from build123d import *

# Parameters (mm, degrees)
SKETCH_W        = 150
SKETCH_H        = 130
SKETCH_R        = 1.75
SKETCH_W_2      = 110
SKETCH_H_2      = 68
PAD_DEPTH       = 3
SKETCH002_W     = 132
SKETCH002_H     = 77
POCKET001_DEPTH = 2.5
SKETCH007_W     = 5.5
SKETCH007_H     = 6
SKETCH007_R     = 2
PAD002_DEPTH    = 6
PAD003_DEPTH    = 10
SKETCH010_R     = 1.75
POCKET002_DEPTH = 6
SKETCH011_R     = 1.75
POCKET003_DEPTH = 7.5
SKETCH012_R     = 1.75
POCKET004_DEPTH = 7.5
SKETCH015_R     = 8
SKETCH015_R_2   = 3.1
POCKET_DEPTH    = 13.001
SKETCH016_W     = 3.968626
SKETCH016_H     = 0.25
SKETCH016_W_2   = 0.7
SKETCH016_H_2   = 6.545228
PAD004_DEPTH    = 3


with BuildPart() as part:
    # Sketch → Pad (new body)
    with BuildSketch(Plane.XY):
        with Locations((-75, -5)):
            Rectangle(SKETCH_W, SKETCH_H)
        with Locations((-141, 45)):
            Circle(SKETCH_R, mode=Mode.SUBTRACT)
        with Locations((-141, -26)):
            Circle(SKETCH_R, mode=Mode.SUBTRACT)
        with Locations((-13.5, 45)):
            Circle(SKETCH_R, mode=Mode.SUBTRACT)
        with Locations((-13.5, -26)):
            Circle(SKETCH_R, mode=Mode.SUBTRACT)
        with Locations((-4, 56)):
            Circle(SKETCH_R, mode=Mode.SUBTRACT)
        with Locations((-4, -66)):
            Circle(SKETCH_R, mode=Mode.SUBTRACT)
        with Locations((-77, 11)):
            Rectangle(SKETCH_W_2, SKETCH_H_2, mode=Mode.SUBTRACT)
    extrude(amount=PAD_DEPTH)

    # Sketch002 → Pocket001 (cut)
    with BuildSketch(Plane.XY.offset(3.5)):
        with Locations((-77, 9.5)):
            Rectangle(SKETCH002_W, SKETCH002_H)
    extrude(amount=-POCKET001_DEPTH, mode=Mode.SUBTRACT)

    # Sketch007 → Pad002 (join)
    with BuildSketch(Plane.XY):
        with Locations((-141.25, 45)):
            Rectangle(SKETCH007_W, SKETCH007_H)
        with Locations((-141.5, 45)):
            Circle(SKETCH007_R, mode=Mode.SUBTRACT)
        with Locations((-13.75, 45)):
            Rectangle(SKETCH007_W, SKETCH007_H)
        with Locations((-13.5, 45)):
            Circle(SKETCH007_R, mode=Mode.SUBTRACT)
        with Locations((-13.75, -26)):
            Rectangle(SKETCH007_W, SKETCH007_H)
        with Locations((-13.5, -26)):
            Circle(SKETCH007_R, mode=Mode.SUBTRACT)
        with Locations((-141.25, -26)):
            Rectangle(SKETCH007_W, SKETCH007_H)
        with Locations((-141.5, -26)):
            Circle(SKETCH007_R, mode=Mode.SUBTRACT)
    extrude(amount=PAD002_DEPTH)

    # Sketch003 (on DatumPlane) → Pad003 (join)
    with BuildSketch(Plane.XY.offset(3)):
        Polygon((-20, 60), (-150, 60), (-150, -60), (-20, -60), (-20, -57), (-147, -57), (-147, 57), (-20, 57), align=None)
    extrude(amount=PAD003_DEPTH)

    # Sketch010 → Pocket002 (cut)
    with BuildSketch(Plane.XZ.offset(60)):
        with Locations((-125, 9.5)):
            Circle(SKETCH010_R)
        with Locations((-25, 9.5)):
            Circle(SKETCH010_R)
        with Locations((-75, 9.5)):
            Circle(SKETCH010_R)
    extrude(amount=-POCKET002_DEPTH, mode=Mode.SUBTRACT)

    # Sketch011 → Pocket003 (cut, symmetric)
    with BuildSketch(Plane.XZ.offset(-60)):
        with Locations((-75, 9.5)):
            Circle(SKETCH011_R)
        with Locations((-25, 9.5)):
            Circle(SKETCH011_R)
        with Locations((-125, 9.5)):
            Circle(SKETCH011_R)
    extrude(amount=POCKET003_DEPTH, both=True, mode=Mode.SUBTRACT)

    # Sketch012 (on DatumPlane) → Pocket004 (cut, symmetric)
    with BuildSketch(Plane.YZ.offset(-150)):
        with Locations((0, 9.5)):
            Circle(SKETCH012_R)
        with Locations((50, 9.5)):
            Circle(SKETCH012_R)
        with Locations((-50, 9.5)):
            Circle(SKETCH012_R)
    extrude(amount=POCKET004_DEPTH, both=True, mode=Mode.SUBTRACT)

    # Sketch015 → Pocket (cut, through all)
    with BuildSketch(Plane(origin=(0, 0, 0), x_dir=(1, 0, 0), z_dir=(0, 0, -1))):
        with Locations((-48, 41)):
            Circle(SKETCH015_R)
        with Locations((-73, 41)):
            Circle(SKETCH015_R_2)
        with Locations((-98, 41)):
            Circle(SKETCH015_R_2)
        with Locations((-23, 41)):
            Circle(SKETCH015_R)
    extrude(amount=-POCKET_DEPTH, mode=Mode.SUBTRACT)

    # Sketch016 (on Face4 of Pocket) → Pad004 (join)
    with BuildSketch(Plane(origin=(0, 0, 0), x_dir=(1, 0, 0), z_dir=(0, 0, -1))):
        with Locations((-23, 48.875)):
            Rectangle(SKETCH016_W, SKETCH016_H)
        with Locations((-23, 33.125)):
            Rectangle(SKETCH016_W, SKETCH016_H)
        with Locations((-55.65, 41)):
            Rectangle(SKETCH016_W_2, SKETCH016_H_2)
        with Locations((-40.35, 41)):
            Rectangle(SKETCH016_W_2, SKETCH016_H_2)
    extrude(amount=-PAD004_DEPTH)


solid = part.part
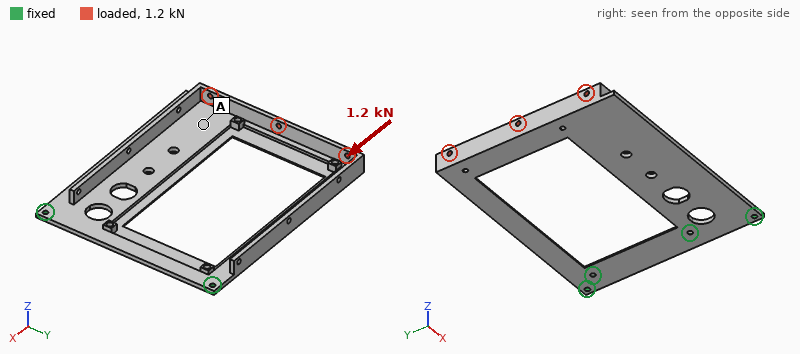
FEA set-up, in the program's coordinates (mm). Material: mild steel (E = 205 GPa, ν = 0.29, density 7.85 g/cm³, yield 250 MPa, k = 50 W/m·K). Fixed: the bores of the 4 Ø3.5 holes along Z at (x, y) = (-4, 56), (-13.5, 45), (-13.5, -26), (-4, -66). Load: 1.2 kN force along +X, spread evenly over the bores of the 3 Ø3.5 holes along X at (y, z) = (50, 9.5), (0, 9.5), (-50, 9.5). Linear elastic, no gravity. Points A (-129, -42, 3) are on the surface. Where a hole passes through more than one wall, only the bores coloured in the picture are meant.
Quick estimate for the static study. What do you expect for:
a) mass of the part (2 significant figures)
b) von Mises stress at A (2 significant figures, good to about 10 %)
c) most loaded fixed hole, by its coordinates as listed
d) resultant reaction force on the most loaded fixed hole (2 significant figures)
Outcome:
320 g
24 MPa
(-4, 56)
870 N
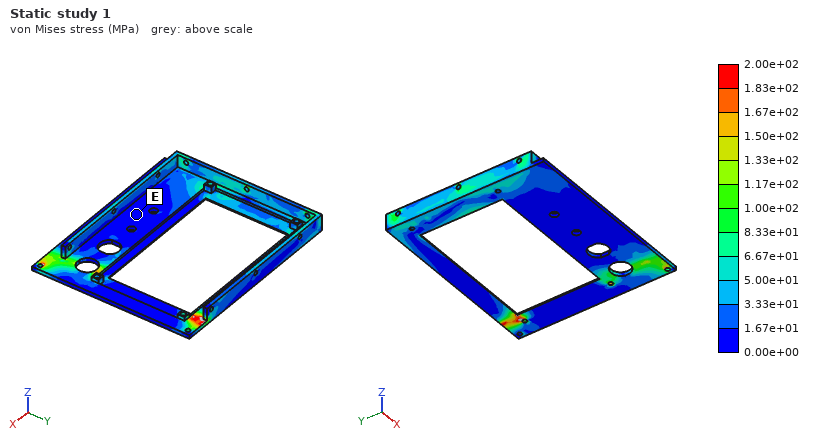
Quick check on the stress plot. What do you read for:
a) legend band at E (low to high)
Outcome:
0.00e+00 to 1.67e+01 MPa
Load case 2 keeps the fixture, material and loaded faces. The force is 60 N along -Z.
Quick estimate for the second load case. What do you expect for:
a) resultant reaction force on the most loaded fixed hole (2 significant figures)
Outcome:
370 N
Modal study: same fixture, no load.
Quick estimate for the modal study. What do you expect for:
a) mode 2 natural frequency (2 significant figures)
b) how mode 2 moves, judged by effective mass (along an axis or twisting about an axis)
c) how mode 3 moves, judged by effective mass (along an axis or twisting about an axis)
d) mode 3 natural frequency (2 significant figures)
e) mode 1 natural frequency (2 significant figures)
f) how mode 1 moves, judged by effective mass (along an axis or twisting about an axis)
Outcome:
230 Hz
twisting about X
along Y
1100 Hz
110 Hz
along Z
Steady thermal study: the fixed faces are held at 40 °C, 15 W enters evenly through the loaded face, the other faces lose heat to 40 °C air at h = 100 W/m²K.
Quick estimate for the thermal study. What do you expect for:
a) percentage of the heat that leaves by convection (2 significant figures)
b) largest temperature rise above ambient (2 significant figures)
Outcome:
100 %
33 K
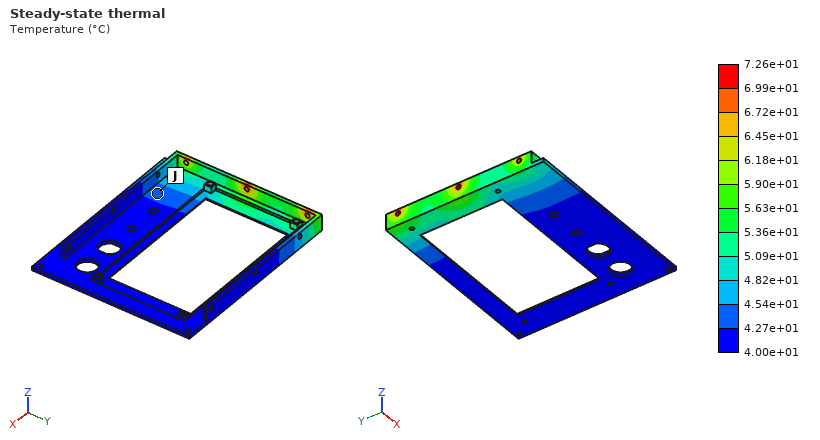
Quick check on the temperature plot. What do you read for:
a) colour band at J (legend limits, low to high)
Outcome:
4.27e+01 to 4.54e+01 °C
